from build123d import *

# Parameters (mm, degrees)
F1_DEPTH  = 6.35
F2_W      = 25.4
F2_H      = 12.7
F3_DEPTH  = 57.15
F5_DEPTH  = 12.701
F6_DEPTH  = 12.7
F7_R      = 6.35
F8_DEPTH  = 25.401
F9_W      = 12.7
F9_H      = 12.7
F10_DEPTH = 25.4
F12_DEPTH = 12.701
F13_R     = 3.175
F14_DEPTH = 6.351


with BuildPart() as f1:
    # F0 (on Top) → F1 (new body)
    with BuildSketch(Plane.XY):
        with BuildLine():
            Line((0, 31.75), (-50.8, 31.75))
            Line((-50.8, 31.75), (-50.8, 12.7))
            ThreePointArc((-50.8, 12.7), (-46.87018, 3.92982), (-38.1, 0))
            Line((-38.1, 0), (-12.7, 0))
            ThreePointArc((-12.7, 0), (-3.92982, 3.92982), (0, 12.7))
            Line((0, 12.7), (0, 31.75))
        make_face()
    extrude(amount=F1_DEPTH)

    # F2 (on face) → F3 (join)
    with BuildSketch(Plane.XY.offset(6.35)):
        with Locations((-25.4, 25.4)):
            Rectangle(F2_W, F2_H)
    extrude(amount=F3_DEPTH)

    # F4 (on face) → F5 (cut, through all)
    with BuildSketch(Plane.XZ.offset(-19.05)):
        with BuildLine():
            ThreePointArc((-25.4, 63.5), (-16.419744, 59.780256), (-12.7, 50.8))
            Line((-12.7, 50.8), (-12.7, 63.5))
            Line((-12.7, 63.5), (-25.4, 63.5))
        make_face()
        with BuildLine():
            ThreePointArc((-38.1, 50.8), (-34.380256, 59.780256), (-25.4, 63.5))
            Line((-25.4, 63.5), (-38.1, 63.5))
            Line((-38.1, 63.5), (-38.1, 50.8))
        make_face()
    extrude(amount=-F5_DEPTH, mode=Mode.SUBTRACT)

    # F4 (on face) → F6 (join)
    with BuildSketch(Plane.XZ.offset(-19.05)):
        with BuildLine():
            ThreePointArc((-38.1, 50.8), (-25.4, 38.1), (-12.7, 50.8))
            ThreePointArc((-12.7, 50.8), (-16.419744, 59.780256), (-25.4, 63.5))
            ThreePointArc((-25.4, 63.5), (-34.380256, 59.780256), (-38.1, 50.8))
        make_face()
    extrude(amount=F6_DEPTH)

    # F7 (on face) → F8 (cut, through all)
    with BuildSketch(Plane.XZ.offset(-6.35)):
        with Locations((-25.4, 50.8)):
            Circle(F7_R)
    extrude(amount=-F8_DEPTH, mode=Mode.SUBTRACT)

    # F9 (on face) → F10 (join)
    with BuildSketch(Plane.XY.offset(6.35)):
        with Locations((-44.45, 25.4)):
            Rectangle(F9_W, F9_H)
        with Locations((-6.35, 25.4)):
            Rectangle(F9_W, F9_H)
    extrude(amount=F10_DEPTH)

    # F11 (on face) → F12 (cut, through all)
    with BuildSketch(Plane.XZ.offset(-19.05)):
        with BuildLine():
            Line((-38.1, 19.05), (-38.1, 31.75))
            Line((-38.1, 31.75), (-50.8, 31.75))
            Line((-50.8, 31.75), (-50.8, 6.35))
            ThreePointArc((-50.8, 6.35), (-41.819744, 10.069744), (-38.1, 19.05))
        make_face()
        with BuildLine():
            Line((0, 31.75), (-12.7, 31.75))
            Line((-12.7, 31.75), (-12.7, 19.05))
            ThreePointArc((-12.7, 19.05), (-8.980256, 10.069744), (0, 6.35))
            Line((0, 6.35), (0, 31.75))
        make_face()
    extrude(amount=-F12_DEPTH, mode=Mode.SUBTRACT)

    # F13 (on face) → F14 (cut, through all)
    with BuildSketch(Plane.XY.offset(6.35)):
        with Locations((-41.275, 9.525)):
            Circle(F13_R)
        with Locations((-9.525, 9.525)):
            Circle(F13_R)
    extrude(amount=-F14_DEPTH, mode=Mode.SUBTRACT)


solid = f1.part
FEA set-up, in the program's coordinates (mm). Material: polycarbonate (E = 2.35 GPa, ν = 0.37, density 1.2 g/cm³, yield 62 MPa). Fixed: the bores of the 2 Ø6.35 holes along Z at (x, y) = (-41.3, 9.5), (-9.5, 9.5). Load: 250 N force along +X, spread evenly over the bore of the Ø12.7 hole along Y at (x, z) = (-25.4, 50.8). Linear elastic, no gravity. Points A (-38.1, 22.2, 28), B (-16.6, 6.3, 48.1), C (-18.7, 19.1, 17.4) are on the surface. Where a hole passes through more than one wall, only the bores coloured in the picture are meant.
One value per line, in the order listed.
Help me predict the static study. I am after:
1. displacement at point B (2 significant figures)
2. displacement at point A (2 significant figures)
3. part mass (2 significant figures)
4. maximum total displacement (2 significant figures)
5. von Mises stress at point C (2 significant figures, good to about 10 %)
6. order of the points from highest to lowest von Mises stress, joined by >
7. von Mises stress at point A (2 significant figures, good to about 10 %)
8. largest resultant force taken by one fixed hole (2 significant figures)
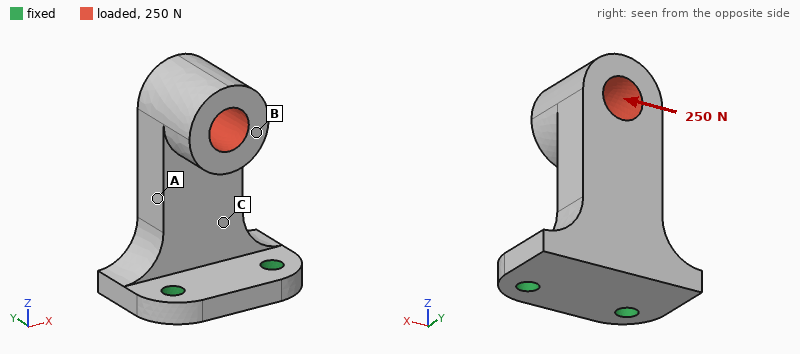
0.74 mm
0.34 mm
37 g
0.94 mm
6.4 MPa
C > A > B
4.9 MPa
380 N
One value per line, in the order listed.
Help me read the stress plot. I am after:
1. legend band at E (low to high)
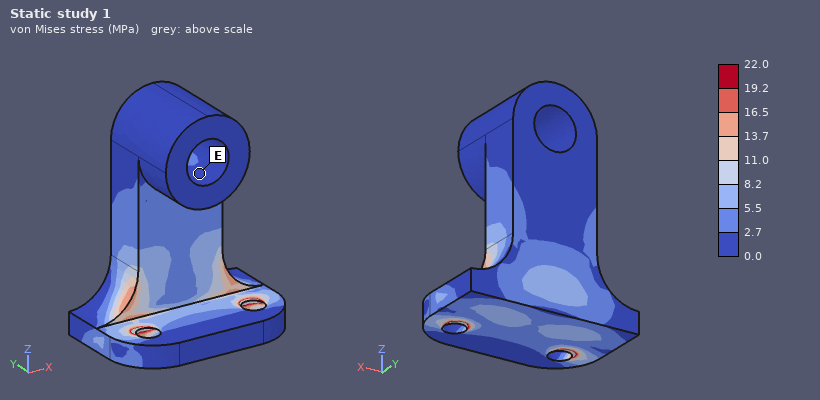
0.0 to 2.7 MPa
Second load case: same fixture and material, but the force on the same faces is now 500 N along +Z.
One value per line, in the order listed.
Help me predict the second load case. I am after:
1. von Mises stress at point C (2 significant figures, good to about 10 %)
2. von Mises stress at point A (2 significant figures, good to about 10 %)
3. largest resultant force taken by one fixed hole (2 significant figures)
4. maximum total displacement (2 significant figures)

5.5 MPa
3.7 MPa
250 N
0.28 mm
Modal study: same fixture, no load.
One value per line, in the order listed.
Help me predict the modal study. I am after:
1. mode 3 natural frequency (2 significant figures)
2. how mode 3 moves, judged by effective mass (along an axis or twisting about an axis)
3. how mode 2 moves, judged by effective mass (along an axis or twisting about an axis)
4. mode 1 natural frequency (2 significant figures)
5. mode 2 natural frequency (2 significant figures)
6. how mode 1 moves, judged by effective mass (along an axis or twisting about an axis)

1700 Hz
along Z
along X
350 Hz
800 Hz
along Y
